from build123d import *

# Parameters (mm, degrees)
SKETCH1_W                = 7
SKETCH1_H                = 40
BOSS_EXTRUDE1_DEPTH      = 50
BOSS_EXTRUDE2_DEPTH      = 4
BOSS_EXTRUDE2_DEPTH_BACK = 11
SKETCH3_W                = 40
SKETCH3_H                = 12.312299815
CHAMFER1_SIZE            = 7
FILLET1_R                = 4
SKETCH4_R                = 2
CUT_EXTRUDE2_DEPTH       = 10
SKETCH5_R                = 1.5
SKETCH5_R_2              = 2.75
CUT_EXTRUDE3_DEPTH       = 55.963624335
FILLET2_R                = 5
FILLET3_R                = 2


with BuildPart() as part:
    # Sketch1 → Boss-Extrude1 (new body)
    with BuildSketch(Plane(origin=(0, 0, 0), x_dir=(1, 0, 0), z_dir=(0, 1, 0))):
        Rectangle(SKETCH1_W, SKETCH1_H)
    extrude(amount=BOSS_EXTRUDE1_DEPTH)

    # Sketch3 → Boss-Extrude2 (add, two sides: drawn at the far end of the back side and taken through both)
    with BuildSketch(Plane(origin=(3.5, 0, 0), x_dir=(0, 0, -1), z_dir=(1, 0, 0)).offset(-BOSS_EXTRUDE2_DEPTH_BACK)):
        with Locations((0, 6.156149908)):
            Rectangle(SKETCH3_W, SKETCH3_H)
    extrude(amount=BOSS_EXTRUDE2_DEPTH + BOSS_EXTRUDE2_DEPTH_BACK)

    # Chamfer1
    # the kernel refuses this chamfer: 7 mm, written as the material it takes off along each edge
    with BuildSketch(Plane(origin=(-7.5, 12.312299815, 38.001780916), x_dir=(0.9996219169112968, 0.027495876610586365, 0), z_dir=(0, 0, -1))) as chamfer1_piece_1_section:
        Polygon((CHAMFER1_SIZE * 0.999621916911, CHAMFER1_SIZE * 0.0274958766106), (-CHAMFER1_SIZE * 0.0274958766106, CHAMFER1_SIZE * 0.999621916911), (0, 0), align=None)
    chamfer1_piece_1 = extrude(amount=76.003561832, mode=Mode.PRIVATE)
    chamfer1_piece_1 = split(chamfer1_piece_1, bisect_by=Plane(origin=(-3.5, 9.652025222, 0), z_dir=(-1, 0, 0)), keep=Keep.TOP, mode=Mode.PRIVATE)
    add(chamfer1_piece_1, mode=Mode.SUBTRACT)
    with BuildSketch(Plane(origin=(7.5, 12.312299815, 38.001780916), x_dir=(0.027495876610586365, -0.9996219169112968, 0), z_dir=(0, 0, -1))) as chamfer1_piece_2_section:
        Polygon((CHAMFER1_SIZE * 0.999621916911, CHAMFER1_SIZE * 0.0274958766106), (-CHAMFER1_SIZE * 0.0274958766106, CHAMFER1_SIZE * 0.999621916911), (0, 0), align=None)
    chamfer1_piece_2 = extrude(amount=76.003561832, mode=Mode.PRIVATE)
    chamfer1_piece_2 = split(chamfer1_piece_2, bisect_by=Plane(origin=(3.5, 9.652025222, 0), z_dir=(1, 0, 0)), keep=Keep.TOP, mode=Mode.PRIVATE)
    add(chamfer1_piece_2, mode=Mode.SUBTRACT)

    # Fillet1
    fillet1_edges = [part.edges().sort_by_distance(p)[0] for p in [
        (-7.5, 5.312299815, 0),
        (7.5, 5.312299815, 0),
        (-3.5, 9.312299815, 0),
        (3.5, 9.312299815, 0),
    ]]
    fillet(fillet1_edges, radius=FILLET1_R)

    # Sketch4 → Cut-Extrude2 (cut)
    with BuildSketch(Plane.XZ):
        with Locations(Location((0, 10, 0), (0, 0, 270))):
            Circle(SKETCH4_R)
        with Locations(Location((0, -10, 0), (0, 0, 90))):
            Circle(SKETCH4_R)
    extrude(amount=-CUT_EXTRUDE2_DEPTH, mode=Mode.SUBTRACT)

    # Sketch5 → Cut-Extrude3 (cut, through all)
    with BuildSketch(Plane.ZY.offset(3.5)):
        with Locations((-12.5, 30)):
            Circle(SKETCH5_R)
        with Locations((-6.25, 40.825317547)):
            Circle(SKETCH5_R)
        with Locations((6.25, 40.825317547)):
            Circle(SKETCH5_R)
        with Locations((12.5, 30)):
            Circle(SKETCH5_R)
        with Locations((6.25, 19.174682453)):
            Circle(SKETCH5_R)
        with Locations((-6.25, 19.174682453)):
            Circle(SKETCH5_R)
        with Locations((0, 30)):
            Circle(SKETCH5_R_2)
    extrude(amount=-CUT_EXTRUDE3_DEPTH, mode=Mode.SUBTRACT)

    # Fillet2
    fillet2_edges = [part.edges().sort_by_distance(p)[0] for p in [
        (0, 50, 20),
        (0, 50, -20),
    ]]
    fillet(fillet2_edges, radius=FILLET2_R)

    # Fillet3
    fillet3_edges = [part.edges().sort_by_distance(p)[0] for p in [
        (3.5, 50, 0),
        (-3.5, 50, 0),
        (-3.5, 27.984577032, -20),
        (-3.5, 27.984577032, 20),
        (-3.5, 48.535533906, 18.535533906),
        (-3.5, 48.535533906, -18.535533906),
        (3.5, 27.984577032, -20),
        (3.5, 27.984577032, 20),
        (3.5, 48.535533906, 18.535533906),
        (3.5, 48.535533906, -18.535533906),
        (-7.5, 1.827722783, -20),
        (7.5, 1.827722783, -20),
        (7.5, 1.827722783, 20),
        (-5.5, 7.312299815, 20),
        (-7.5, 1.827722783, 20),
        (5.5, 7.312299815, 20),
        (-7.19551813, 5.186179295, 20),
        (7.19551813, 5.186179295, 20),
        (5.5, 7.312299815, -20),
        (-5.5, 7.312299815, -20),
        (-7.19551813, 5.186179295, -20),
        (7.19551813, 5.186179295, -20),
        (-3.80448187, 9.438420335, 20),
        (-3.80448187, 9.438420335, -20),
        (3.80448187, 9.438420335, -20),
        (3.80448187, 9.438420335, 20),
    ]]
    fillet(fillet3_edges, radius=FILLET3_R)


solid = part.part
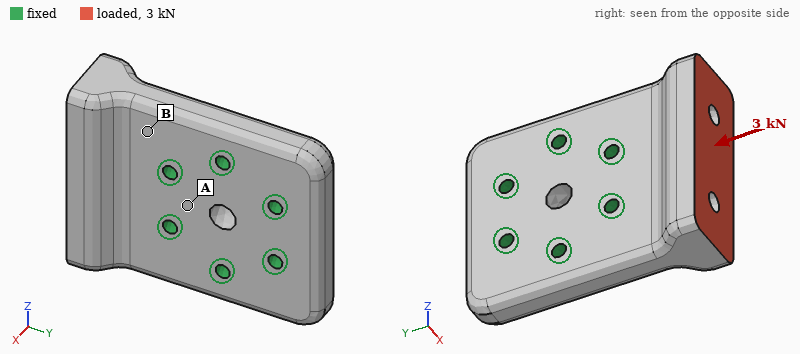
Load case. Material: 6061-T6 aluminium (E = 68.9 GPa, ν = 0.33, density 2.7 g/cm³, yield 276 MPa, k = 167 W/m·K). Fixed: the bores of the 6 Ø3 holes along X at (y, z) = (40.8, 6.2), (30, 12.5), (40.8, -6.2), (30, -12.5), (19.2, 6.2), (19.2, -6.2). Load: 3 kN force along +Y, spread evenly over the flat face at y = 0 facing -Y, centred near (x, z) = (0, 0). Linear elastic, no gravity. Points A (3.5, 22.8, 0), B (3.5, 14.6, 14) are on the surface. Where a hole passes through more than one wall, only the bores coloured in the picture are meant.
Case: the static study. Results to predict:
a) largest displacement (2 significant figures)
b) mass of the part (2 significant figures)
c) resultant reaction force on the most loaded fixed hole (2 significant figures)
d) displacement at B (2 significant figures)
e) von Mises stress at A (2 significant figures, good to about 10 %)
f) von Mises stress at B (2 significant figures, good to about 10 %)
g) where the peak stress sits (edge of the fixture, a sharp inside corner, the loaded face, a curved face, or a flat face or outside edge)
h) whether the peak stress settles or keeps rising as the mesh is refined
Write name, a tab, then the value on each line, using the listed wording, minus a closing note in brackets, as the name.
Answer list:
largest displacement	3.8 µm
mass of the part	41 g
resultant reaction force on the most loaded fixed hole	1.0 kN
displacement at B	1.8 µm
von Mises stress at A	3.8 MPa
von Mises stress at B	8.6 MPa
where the peak stress sits	edge of the fixture
whether the peak stress settles or keeps rising as the mesh is refined	keeps rising
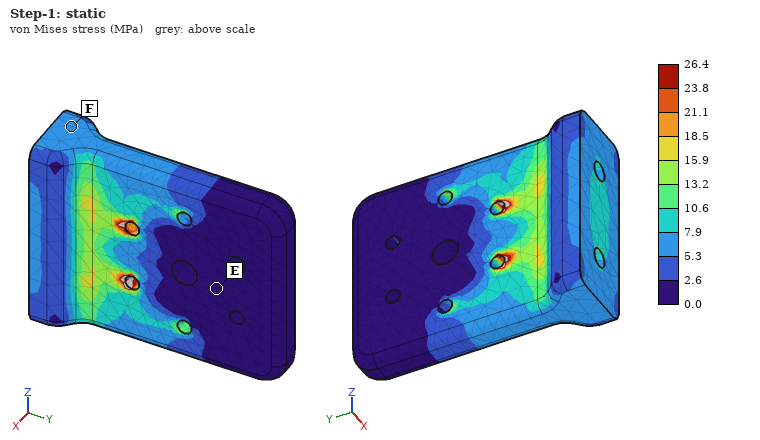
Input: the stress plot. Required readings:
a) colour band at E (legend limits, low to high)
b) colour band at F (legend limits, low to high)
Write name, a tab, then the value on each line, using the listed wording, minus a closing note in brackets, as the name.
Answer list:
colour band at E	0.0 to 2.6 MPa
colour band at F	5.3 to 7.9 MPa
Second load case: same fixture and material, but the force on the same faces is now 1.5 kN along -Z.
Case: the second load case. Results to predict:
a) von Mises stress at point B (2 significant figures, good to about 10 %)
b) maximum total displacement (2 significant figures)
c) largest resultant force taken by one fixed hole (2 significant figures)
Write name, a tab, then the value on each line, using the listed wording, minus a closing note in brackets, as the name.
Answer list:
von Mises stress at point B	9.1 MPa
maximum total displacement	10.0 µm
largest resultant force taken by one fixed hole	1.1 kN
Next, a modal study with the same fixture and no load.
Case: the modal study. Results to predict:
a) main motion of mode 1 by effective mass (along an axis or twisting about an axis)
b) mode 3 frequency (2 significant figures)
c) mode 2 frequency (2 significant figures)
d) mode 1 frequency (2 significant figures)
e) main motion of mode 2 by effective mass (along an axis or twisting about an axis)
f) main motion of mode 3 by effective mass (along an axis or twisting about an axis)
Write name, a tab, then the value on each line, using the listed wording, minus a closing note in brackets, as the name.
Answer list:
main motion of mode 1 by effective mass	along X
mode 3 frequency	21 kHz
mode 2 frequency	13 kHz
mode 1 frequency	9000 Hz
main motion of mode 2 by effective mass	twisting about Y
main motion of mode 3 by effective mass	along Z
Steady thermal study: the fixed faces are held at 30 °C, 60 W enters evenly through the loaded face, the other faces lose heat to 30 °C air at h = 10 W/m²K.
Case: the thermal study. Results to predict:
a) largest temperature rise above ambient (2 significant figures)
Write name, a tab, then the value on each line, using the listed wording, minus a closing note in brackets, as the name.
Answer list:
largest temperature rise above ambient	24 K
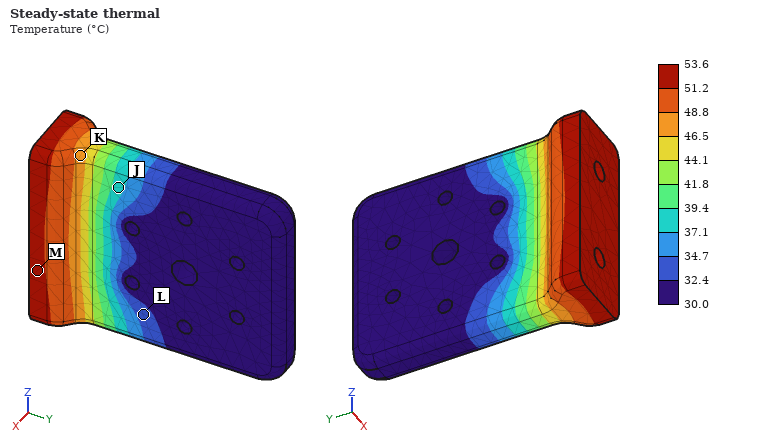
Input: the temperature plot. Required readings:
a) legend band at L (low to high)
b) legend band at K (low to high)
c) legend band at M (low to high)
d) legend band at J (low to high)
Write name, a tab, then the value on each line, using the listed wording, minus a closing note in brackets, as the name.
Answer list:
legend band at L	32.4 to 34.7 °C
legend band at K	46.5 to 48.8 °C
legend band at M	51.2 to 53.6 °C
legend band at J	37.1 to 39.4 °C
